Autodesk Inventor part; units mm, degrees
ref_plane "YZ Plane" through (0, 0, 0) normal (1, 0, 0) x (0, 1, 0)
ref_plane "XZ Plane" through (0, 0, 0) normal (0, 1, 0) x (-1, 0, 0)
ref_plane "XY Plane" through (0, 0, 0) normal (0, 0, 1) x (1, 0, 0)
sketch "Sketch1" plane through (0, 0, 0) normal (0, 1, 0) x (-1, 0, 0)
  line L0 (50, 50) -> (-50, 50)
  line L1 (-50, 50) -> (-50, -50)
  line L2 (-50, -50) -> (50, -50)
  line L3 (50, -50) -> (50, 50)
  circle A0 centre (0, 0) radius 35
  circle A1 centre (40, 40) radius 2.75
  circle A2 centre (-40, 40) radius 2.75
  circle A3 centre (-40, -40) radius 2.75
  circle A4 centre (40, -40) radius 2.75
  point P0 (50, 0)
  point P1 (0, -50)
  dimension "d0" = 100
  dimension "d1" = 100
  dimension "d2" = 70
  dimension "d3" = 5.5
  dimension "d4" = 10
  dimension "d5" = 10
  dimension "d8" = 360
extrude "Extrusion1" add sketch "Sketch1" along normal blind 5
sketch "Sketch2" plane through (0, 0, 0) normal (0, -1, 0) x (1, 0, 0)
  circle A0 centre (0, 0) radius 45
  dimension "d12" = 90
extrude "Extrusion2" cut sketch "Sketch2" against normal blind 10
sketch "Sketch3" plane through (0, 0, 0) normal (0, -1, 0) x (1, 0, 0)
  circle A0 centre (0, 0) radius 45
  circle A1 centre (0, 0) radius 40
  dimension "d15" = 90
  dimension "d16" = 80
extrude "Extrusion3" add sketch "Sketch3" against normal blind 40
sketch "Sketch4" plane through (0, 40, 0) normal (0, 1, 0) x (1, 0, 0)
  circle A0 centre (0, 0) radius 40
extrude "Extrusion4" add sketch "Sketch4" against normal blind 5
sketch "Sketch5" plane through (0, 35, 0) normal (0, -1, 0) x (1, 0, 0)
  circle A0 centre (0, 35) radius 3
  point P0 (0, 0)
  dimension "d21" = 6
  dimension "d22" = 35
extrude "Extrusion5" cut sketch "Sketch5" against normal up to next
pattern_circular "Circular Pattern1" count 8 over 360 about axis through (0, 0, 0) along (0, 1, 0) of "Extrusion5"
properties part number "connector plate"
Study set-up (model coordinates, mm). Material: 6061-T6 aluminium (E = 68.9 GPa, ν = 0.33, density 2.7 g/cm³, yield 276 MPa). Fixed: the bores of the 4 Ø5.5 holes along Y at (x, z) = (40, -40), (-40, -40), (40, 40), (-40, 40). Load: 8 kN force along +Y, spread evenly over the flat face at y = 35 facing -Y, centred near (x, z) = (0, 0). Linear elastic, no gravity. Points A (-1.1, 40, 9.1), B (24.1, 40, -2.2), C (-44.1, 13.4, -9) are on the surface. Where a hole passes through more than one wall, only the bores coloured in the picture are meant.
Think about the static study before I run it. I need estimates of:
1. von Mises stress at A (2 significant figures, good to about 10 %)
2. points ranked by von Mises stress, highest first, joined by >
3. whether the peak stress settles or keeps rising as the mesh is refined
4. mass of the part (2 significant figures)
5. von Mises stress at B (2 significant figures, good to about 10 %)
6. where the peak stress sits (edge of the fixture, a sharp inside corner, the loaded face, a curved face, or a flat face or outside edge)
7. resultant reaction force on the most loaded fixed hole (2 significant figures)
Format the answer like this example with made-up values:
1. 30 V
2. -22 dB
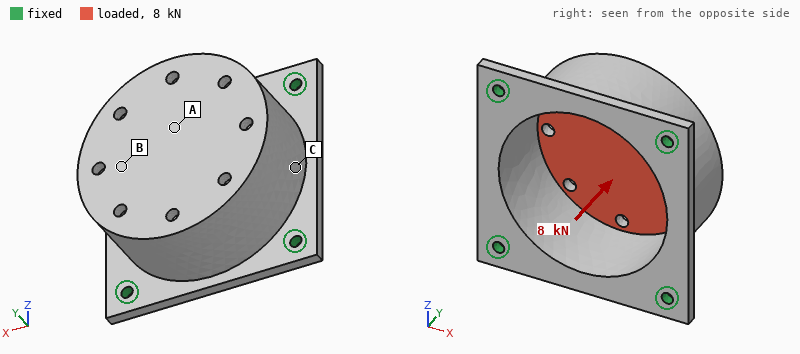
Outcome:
1. 71 MPa
2. A > B > C
3. keeps rising
4. 260 g
5. 43 MPa
6. edge of the fixture
7. 2.2 kN
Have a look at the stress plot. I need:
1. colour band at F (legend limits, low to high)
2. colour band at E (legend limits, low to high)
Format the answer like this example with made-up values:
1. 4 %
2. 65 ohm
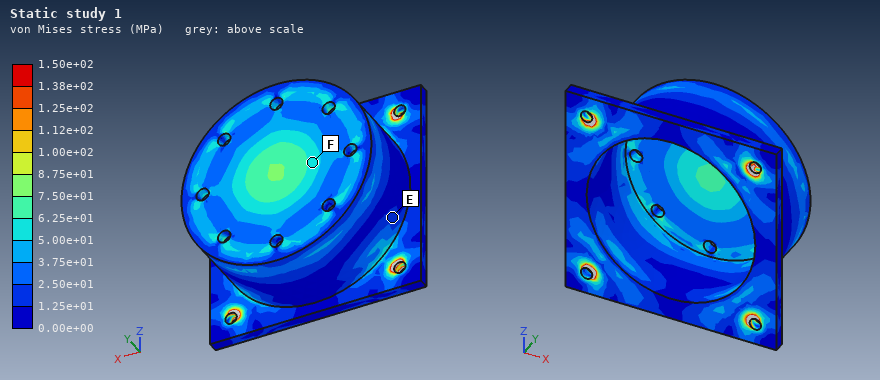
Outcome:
1. 5.00e+01 to 6.25e+01 MPa
2. 1.25e+01 to 2.50e+01 MPa
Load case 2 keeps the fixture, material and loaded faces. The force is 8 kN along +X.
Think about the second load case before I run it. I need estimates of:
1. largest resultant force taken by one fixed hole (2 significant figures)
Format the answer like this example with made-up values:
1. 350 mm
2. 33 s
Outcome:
1. 2.7 kN
